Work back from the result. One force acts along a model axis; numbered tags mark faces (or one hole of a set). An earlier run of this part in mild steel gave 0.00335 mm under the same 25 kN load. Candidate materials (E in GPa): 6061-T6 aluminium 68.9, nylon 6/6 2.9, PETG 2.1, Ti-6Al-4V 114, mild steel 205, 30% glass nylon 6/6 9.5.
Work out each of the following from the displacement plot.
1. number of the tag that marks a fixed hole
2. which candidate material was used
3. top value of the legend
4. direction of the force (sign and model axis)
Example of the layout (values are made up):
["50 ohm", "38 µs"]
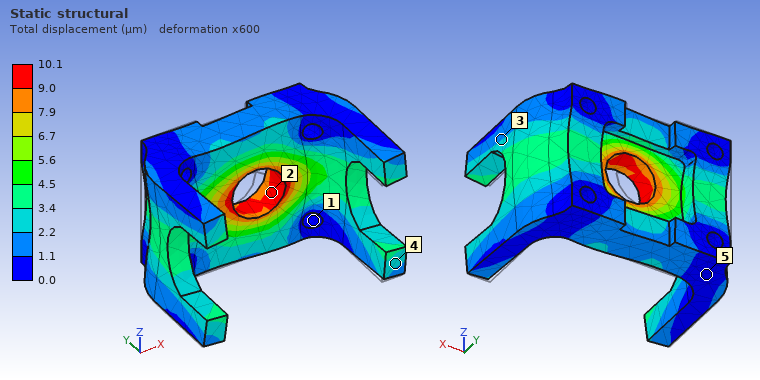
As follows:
["1", "6061-T6 aluminium", "10.1 µm", "+X"]
